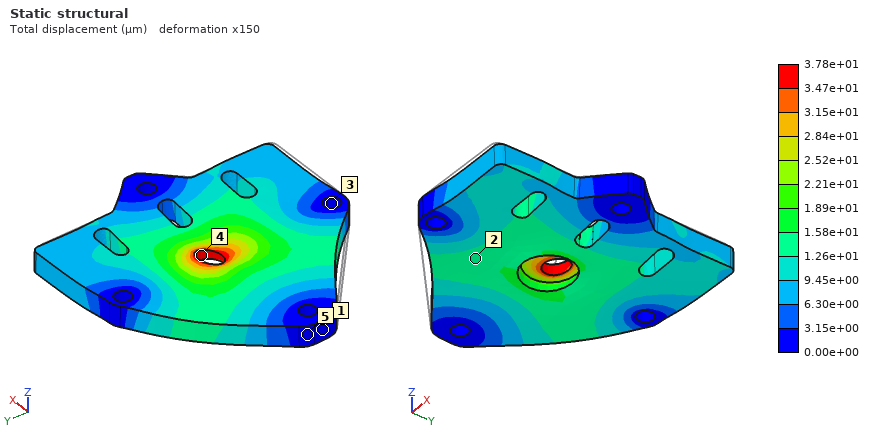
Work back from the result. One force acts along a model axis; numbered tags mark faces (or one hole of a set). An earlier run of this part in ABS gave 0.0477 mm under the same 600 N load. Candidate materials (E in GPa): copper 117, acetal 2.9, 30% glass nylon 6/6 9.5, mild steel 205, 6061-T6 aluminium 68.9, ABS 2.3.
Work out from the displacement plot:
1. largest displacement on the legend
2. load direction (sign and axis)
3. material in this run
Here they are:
3.78e+01 µm
+Y
acetal
